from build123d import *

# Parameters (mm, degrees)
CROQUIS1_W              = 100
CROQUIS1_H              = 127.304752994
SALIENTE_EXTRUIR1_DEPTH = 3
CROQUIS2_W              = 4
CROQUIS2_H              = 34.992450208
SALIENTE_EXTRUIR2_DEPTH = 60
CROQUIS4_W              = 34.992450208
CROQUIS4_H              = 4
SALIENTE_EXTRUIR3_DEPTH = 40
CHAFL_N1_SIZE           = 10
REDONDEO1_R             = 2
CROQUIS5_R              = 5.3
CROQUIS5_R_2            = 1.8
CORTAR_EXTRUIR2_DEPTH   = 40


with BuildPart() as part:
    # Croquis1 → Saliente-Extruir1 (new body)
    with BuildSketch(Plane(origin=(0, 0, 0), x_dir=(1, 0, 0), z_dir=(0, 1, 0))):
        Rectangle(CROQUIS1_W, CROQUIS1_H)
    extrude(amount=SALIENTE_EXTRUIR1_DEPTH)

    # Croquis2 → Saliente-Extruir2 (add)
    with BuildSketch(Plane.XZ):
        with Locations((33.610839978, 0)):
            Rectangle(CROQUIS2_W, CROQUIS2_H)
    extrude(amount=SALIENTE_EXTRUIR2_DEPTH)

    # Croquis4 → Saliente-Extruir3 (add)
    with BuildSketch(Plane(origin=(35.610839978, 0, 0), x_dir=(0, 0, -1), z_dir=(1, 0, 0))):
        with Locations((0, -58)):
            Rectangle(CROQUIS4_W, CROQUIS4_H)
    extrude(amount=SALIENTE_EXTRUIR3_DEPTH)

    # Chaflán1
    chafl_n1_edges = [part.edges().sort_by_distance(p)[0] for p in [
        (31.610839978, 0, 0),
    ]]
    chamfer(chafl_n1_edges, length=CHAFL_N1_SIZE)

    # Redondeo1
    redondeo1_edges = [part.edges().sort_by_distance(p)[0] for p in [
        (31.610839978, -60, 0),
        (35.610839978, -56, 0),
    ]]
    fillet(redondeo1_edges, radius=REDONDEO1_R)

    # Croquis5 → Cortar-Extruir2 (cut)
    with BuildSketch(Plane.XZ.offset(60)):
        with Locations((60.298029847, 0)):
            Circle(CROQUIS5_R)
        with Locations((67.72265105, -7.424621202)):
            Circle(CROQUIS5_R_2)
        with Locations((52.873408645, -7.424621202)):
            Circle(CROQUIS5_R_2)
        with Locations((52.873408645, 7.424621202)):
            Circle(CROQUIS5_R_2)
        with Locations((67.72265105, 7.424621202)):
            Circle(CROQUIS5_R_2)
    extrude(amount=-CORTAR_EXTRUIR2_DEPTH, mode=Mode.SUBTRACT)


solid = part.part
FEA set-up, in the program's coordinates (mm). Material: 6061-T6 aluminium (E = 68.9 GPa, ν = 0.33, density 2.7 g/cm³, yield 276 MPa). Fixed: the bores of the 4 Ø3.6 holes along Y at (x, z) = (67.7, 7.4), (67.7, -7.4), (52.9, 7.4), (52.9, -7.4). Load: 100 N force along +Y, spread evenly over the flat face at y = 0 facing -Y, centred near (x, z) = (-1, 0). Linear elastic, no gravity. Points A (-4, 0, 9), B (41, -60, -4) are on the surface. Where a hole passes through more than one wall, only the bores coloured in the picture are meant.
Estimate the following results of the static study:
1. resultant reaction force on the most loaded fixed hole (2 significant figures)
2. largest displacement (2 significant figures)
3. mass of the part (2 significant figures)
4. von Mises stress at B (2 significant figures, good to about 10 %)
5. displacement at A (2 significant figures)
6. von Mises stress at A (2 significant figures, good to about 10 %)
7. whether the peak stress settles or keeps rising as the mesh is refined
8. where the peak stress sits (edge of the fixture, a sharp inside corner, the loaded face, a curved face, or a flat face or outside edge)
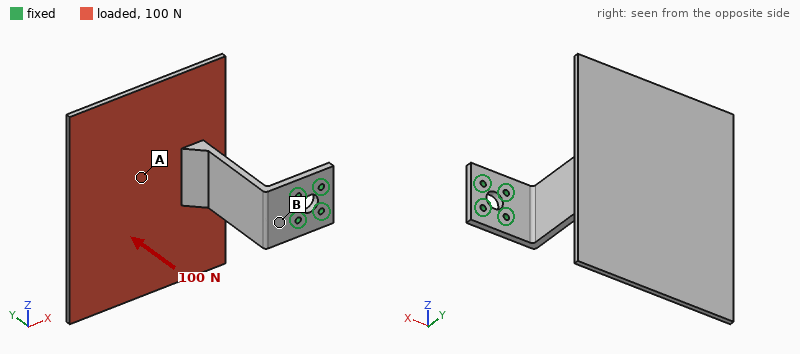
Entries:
92 N
2.1 mm
140 g
40 MPa
1.1 mm
6.9 MPa
keeps rising
edge of the fixture
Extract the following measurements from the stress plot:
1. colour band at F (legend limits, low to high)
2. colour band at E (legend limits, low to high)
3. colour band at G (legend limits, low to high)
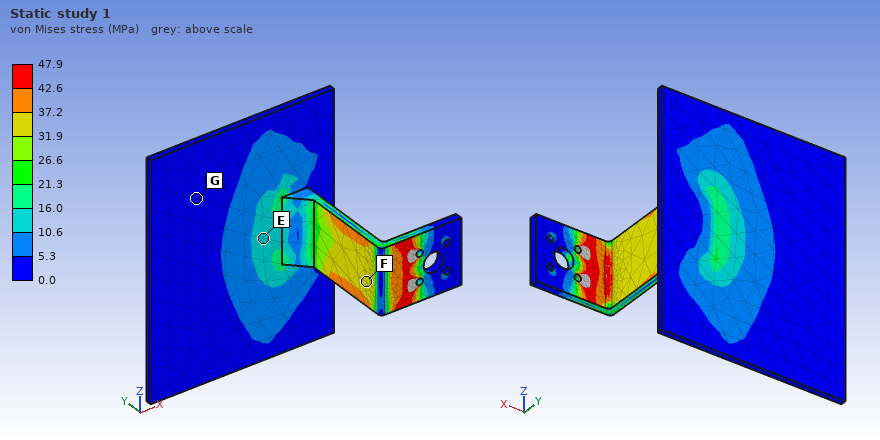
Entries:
31.9 to 37.2 MPa
10.6 to 16.0 MPa
0.0 to 5.3 MPa
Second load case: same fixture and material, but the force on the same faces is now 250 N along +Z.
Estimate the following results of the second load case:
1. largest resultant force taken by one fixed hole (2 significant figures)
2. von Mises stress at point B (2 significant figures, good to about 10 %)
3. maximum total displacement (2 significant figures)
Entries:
930 N
55 MPa
2.0 mm
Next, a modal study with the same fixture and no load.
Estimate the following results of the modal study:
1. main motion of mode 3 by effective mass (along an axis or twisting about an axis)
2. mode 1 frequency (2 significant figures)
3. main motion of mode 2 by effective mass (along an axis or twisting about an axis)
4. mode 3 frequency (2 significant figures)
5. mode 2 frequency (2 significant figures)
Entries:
along Z
110 Hz
along Z
310 Hz
190 Hz
